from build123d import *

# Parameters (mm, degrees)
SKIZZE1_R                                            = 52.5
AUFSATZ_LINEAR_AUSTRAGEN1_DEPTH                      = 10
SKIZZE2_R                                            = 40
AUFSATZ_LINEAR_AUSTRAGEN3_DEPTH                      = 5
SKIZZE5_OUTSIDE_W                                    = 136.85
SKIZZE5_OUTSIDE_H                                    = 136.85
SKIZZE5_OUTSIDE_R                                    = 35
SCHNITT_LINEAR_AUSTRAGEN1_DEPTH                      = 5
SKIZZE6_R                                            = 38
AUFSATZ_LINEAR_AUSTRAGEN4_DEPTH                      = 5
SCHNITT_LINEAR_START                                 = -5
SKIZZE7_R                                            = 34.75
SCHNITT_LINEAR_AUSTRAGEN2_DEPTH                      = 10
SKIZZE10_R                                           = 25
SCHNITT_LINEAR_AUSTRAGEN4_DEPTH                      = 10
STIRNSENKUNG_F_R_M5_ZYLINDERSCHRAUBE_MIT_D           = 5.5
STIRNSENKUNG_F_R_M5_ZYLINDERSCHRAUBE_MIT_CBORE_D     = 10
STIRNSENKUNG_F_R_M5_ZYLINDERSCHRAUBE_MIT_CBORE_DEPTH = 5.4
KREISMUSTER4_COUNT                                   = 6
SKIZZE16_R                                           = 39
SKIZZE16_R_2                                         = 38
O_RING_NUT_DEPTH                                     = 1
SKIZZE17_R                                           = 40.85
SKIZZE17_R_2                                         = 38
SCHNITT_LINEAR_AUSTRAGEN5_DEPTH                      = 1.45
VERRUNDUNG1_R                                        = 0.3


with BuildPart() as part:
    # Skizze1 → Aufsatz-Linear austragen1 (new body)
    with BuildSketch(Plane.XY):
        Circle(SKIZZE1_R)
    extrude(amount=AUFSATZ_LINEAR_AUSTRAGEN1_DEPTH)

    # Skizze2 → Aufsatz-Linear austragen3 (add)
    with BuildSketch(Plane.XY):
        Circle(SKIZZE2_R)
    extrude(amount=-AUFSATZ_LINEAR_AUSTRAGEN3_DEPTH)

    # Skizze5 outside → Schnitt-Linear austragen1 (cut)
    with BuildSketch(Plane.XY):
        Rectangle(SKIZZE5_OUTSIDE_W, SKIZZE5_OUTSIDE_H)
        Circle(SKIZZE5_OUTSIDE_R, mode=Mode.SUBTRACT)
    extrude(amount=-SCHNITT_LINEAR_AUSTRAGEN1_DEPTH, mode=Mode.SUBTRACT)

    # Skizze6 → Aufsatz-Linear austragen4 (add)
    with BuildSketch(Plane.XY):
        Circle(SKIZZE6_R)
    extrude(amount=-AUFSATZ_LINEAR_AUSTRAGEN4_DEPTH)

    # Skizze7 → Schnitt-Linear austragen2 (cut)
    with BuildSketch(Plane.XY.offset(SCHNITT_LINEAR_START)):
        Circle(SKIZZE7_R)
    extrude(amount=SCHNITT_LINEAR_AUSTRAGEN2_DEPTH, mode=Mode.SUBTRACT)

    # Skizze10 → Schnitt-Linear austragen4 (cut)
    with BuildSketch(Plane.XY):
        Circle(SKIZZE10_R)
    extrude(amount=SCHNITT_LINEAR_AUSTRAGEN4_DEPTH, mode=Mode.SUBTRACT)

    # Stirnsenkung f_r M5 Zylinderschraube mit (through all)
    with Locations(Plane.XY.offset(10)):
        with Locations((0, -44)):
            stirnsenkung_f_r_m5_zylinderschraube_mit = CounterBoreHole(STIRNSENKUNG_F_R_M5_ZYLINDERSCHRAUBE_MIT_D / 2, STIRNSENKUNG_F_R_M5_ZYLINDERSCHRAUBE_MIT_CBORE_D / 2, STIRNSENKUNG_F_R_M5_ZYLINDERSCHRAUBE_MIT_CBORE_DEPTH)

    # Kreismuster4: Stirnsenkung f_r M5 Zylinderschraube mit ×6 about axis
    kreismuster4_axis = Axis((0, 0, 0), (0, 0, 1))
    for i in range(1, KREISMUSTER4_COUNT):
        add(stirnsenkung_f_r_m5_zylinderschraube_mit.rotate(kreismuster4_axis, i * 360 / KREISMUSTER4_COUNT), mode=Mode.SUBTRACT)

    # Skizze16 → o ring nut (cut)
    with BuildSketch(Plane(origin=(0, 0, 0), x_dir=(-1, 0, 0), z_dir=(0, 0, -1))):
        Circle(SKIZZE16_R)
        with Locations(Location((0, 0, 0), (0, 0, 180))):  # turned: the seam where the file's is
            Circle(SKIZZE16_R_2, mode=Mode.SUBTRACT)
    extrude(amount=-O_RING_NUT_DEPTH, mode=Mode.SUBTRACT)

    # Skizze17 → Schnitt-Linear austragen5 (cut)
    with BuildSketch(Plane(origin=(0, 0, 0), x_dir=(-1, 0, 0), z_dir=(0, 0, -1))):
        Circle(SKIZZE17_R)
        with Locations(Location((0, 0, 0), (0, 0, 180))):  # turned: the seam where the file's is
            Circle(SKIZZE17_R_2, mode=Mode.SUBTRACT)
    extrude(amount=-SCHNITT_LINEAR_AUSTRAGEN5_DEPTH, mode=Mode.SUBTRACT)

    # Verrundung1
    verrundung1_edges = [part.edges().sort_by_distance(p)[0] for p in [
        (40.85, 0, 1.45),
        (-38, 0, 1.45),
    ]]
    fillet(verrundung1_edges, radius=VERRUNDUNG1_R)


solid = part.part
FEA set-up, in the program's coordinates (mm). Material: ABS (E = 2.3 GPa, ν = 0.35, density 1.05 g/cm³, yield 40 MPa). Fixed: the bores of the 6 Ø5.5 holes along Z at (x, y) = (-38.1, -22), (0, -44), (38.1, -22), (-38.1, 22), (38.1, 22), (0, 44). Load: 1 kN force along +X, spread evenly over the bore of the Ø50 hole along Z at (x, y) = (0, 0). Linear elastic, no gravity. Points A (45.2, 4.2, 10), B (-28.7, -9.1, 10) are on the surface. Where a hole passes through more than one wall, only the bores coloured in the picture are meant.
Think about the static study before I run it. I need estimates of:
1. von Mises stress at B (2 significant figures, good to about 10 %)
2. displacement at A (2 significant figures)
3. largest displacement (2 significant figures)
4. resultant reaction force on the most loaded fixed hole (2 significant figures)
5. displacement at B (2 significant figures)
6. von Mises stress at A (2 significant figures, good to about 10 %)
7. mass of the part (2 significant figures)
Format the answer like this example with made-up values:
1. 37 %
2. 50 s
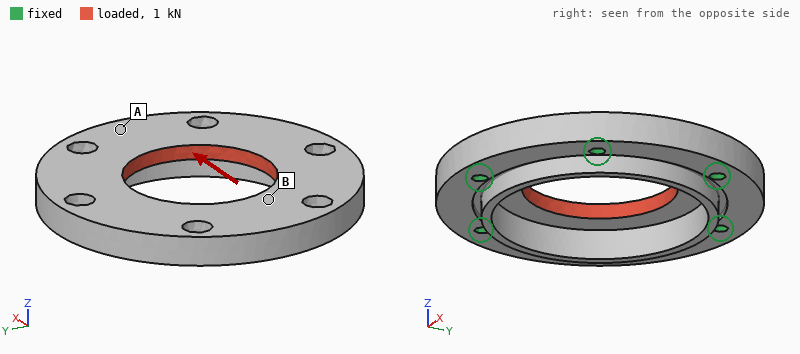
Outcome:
1. 1.8 MPa
2. 32 µm
3. 59 µm
4. 180 N
5. 45 µm
6. 0.72 MPa
7. 60 g
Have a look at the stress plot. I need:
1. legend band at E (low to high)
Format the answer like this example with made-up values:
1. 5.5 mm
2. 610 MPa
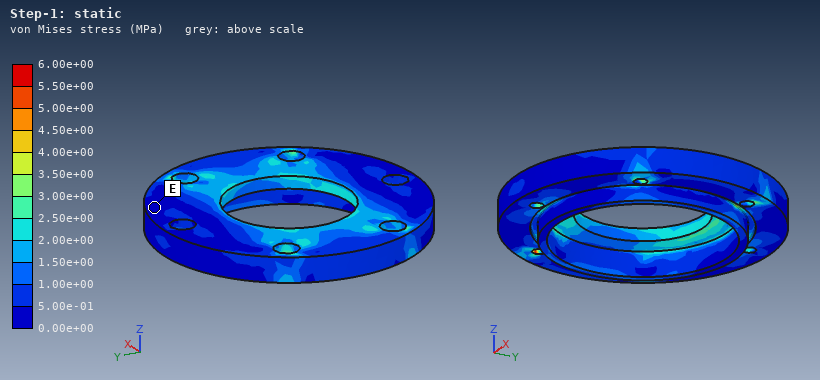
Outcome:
1. 0.00e+00 to 5.00e-01 MPa
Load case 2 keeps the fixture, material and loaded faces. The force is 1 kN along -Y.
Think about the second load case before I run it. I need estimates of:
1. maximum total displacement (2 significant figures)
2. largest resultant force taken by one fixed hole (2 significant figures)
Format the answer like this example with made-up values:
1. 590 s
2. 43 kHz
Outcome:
1. 59 µm
2. 180 N
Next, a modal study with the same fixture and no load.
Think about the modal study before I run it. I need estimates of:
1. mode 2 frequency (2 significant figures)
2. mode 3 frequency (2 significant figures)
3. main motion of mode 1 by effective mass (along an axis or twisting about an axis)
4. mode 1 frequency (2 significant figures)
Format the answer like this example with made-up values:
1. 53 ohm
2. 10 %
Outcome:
1. 3900 Hz
2. 4000 Hz
3. along Z
4. 3600 Hz
